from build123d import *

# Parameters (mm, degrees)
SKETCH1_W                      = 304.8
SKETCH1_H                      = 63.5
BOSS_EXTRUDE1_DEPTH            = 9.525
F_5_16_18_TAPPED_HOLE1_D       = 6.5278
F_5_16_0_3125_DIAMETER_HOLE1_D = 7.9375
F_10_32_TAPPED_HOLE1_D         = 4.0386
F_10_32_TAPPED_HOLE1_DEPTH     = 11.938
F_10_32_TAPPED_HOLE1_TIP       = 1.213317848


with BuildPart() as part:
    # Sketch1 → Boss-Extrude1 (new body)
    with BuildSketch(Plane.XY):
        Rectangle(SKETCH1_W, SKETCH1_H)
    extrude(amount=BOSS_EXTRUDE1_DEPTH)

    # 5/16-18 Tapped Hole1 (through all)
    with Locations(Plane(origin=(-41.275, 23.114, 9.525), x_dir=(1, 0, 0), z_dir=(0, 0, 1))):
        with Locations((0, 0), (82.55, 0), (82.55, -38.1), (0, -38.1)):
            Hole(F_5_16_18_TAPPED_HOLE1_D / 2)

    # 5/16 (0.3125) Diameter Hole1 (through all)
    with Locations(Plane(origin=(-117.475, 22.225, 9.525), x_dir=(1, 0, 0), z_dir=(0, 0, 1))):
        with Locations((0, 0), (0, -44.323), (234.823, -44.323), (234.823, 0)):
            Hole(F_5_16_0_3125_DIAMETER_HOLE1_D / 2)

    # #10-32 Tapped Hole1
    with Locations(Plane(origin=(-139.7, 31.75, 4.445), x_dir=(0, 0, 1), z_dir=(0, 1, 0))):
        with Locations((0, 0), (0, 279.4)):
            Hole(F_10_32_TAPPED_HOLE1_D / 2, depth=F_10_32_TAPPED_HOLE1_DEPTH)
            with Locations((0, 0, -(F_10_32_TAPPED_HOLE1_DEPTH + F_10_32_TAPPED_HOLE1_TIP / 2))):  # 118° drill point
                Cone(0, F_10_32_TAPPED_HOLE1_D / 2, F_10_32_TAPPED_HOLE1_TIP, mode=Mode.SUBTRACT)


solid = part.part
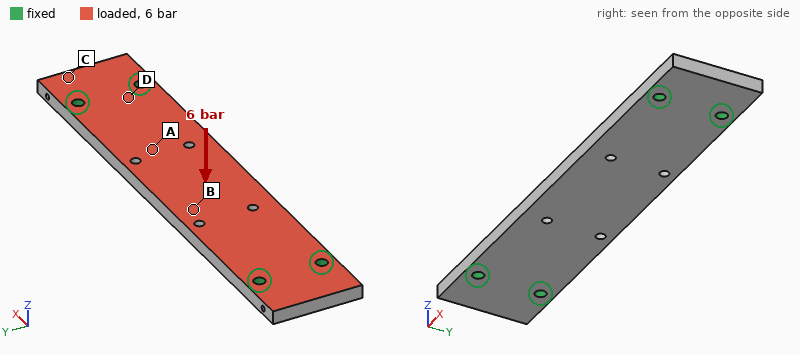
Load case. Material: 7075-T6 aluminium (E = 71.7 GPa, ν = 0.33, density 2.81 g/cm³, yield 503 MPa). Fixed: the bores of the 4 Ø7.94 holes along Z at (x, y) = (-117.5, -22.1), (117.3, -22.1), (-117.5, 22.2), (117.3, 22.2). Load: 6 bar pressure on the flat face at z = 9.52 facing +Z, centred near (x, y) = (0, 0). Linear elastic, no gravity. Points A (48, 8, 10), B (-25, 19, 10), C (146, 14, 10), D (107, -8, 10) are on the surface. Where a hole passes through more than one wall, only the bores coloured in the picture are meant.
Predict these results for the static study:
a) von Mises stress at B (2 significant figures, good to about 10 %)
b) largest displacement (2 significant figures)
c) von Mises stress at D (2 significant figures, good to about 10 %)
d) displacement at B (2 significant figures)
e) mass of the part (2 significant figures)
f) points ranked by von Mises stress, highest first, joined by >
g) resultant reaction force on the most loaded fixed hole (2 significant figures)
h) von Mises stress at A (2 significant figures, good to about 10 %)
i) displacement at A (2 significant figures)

74 MPa
0.93 mm
100 MPa
0.83 mm
510 g
D > B > A > C
2.9 kN
46 MPa
0.64 mm
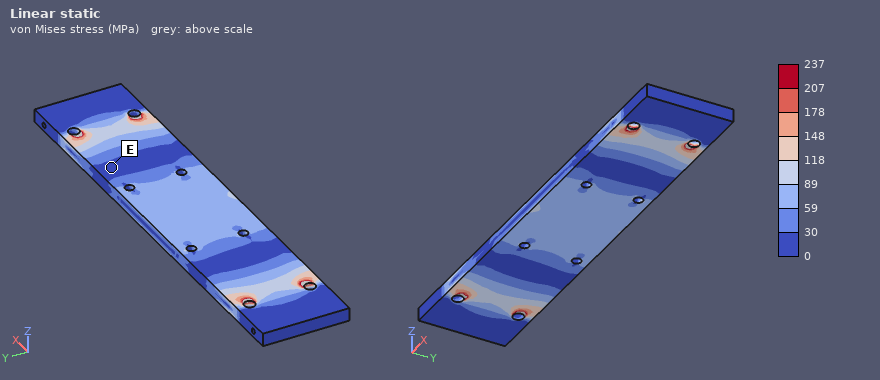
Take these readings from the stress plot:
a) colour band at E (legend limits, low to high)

0 to 30 MPa
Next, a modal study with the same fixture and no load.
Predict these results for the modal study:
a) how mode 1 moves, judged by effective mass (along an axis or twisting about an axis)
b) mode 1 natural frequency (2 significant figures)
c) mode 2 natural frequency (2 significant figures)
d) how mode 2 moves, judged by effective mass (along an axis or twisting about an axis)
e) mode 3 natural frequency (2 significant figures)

along Z
900 Hz
2200 Hz
twisting about X
2400 Hz
